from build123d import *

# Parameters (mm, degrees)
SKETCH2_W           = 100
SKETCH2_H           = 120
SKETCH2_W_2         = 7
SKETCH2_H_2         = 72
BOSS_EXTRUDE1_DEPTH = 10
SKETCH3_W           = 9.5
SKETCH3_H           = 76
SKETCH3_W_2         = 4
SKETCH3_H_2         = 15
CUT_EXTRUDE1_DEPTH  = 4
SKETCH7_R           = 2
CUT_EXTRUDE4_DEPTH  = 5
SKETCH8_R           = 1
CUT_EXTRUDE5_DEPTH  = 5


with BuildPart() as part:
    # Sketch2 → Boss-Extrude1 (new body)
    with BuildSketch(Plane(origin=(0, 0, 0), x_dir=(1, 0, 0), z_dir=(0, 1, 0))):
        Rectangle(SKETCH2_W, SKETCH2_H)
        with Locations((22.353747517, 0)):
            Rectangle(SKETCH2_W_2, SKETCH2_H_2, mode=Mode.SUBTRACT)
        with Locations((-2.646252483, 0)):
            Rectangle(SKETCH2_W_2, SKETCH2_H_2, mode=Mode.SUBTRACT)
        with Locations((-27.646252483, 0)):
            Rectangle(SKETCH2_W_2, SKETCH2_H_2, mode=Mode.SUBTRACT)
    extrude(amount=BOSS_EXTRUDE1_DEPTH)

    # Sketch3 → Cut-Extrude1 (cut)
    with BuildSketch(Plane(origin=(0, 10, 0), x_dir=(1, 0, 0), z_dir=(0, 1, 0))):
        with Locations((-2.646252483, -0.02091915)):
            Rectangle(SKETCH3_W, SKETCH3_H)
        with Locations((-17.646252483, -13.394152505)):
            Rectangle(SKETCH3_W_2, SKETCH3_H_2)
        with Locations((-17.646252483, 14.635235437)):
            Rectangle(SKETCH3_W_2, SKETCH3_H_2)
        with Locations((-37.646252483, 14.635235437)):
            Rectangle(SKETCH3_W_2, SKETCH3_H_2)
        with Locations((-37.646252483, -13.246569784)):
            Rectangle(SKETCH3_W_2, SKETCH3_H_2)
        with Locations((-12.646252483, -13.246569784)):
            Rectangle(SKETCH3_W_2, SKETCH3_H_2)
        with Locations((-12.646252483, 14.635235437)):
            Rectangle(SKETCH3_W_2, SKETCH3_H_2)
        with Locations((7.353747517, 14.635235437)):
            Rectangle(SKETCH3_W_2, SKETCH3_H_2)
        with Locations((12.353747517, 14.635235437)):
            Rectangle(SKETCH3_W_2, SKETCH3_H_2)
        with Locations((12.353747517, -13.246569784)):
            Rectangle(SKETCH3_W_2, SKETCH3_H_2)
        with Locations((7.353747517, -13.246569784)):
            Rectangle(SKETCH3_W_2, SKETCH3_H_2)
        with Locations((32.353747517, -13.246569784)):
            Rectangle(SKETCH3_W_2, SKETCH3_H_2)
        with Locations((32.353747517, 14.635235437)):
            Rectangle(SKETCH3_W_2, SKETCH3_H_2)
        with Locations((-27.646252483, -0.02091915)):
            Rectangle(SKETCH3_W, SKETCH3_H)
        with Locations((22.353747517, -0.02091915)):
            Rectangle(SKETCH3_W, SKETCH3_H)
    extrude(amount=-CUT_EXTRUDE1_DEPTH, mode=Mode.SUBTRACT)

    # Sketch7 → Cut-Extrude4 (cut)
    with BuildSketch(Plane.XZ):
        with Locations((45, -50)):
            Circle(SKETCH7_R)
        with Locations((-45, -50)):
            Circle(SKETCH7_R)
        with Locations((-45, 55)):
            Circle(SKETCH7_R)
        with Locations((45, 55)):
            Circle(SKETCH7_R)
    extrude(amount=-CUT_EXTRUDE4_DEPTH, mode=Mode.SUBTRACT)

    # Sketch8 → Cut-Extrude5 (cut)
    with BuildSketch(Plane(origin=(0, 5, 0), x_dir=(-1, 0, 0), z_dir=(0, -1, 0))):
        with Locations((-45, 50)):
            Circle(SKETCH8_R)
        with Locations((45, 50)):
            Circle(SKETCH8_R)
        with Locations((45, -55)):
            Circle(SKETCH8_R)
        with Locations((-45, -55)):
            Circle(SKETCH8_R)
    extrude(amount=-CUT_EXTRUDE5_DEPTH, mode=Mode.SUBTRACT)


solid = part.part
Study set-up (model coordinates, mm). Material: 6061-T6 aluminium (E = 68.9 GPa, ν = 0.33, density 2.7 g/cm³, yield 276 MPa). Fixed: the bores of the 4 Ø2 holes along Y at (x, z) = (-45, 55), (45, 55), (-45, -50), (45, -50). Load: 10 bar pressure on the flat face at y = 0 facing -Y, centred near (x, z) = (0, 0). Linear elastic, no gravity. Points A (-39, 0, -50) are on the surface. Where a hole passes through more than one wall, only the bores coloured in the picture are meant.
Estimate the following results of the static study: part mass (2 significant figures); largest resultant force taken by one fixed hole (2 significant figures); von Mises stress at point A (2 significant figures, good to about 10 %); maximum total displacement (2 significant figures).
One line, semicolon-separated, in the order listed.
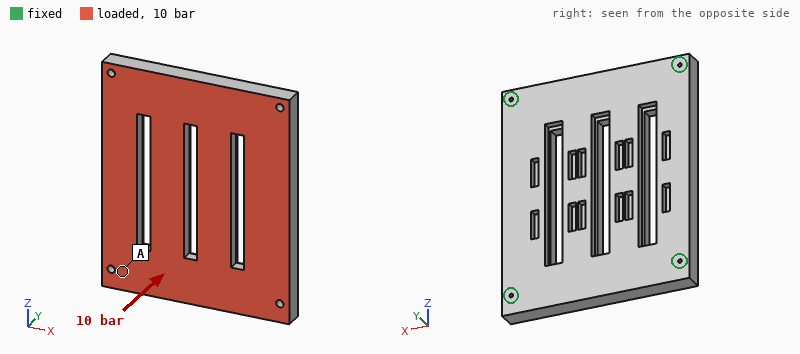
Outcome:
270 g; 4.7 kN; 37 MPa; 0.38 mm
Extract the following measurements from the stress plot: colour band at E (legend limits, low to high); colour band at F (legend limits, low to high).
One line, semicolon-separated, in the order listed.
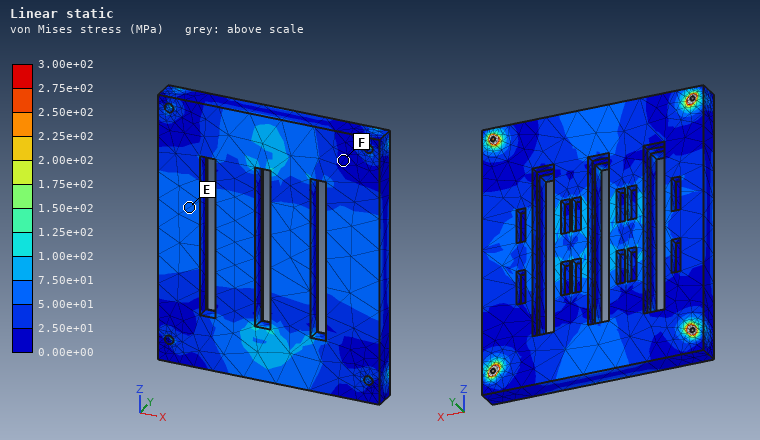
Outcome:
5.00e+01 to 7.50e+01 MPa; 0.00e+00 to 2.50e+01 MPa
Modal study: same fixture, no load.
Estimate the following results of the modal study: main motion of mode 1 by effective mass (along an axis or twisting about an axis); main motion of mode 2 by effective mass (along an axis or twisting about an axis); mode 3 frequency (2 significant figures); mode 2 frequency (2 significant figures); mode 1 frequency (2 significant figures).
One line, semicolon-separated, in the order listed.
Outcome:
along Y; twisting about Z; 3700 Hz; 3400 Hz; 2100 Hz
